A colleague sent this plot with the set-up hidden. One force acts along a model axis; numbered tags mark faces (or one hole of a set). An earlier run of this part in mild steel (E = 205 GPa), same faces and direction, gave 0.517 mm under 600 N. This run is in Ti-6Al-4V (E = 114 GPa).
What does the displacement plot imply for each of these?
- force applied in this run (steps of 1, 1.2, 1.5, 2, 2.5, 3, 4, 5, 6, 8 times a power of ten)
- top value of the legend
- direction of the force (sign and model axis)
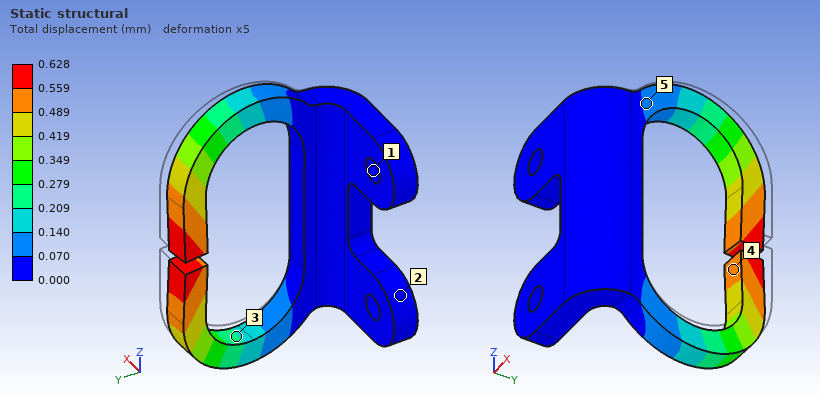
400 N
0.628 mm
-X
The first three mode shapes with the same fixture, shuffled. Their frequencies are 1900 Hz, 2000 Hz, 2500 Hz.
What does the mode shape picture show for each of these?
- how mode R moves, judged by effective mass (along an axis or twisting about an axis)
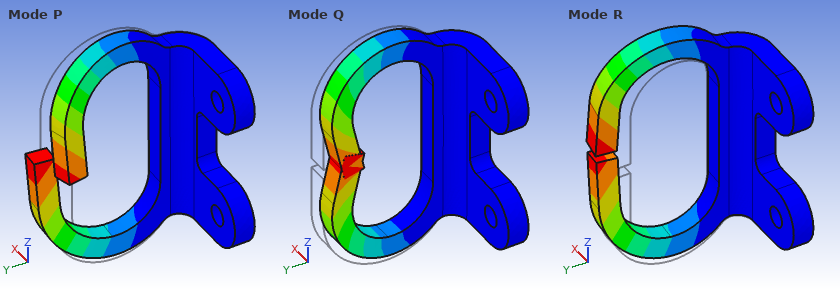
along X
